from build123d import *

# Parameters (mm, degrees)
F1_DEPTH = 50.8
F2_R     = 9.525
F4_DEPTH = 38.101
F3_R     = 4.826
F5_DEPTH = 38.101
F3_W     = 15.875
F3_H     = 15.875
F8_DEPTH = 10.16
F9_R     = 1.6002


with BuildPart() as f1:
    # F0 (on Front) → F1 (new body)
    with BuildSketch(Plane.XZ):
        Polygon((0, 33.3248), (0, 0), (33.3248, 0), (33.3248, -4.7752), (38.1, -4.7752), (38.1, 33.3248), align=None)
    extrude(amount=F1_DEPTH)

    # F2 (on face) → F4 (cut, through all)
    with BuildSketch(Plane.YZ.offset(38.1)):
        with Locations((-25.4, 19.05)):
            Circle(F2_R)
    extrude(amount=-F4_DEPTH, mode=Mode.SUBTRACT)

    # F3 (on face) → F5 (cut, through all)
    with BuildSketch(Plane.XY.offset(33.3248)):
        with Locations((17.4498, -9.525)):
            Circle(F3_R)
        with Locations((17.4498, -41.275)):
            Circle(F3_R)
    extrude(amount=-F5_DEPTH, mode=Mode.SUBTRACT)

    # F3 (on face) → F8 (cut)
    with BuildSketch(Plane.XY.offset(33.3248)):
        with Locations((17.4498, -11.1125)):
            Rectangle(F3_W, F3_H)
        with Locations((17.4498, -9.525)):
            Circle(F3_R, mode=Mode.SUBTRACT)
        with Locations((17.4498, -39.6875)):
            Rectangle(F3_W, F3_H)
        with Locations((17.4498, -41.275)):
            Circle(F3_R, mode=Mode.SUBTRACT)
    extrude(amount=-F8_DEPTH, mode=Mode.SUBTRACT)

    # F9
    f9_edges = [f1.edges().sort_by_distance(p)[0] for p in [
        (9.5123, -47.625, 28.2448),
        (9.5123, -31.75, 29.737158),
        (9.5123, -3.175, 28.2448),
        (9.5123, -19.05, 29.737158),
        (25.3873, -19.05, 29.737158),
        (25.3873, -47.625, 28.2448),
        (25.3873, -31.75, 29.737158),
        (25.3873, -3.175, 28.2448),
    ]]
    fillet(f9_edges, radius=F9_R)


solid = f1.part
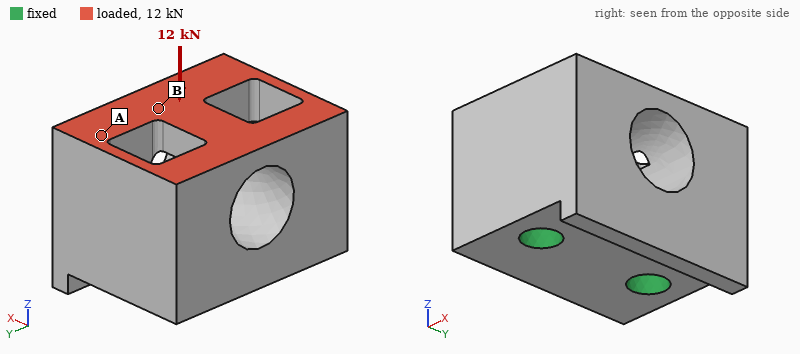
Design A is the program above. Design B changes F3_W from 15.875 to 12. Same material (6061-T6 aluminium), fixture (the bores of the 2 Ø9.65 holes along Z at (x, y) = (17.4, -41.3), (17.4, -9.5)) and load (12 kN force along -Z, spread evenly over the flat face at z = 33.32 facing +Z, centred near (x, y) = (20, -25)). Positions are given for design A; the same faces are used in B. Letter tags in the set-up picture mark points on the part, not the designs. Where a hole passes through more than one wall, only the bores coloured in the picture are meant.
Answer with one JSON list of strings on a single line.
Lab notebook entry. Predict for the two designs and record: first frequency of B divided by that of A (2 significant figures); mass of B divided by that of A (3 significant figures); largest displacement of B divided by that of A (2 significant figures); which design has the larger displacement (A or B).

["1.0", "1.03", "0.67", "A"]
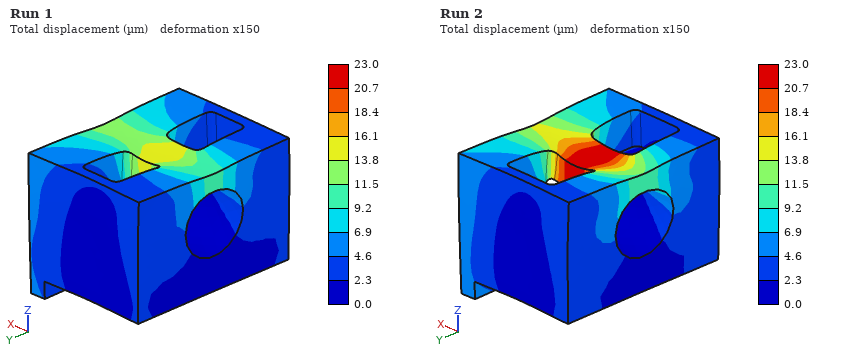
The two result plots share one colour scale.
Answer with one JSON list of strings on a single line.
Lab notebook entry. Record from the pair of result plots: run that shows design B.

["Run 1"]
